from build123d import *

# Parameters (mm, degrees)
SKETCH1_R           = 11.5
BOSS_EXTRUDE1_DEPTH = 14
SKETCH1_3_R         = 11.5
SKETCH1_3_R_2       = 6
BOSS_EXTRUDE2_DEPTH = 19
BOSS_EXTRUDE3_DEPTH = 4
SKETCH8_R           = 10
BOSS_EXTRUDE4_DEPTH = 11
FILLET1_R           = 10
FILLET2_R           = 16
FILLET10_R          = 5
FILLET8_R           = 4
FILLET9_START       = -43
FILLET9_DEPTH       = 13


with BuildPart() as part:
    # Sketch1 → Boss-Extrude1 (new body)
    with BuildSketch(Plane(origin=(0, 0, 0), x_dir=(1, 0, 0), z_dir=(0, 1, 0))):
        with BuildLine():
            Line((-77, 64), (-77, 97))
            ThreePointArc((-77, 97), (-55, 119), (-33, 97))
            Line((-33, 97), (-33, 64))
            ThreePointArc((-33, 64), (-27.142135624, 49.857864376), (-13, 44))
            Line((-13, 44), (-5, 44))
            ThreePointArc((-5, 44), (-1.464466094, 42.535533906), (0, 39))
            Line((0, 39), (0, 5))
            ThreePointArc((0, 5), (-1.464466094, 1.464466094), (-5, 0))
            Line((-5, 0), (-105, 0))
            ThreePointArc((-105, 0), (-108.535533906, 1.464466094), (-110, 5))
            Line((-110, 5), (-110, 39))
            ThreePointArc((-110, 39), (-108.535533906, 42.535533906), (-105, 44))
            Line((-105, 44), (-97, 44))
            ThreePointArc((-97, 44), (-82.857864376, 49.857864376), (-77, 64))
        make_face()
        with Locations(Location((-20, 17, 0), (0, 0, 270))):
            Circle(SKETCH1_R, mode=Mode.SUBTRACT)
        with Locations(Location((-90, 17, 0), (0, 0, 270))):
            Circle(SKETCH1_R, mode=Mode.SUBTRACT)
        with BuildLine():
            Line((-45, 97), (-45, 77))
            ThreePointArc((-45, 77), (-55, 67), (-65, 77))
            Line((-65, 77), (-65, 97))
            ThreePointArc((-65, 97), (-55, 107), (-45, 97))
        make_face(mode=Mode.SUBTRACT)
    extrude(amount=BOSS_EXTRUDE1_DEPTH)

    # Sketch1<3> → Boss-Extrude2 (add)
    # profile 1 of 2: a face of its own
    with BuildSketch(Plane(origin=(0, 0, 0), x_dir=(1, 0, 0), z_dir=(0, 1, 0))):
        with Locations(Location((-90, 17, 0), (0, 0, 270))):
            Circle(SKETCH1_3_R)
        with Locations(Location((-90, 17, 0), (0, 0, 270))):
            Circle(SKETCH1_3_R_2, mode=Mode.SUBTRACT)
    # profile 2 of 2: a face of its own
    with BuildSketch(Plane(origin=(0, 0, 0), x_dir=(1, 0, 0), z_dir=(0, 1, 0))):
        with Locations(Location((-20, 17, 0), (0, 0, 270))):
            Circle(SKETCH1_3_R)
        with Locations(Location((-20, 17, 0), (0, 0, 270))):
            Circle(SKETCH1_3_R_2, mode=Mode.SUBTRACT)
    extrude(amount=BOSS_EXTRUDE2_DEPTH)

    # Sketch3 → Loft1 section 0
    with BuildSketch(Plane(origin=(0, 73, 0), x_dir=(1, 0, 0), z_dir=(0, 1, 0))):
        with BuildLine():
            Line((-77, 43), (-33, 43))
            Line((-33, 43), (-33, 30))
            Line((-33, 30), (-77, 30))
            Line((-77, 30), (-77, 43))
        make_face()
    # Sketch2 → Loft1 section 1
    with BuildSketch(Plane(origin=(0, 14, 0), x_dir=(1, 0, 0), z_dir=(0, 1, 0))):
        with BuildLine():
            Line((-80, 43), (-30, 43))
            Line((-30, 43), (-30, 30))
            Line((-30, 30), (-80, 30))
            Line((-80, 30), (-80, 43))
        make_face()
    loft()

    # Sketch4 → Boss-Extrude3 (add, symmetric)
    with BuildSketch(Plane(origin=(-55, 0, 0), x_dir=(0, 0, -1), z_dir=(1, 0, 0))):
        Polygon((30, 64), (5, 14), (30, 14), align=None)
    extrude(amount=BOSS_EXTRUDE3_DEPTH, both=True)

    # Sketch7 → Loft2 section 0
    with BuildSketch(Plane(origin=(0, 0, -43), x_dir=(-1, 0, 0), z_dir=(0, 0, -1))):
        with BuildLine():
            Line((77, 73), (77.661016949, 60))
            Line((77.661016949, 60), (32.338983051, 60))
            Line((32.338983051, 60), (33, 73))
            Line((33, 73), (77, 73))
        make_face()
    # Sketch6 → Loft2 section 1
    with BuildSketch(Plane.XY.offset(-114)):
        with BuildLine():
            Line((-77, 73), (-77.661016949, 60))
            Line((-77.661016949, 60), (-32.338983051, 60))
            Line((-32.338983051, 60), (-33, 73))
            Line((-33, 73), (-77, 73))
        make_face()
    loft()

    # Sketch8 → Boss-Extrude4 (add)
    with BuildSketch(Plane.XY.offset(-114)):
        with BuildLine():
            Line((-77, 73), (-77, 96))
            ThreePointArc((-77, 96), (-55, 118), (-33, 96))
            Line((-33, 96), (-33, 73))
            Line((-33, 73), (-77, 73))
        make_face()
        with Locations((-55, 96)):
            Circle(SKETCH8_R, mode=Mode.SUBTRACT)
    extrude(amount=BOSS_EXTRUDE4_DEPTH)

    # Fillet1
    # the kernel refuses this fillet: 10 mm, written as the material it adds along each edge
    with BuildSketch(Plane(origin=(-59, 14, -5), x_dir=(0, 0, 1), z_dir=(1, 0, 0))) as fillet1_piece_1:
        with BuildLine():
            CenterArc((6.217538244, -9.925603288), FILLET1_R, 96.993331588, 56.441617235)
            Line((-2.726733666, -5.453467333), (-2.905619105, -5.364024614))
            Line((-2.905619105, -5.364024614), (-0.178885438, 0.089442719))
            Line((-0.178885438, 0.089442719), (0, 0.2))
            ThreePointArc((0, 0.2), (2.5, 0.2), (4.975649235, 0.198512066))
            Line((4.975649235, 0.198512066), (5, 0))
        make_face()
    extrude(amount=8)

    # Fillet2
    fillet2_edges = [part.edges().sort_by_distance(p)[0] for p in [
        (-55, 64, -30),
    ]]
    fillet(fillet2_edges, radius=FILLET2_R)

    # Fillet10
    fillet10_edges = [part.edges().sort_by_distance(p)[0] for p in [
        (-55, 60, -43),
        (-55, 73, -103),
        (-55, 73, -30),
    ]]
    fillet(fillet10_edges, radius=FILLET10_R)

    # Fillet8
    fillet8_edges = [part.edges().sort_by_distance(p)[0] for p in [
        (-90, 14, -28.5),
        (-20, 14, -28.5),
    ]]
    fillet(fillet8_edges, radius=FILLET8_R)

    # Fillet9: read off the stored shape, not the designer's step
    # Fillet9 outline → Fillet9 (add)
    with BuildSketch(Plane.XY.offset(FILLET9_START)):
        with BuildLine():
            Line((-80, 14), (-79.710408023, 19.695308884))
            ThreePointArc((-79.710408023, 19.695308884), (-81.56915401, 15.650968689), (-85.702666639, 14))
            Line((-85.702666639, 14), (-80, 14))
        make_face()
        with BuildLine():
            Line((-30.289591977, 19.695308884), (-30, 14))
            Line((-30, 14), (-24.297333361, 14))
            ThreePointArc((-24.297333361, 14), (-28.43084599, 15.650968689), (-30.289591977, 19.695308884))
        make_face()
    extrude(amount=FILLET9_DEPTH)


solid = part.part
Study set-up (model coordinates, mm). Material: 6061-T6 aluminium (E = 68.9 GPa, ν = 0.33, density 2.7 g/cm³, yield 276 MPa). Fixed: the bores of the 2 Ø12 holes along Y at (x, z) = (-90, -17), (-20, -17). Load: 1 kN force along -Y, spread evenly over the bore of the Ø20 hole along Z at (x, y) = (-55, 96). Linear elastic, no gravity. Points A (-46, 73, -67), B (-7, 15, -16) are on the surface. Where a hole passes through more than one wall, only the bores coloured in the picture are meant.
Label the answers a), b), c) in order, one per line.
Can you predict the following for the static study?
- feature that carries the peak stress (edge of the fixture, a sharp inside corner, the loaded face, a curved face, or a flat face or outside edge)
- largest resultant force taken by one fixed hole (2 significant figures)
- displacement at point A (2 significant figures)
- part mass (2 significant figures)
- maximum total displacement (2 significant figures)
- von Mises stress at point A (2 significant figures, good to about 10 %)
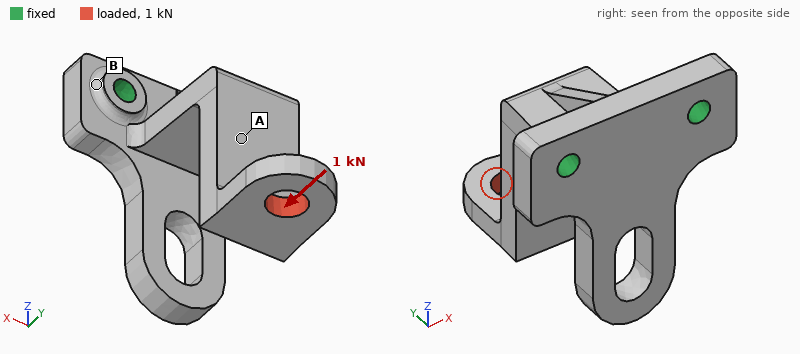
a) a curved face
b) 550 N
c) 0.22 mm
d) 550 g
e) 0.71 mm
f) 32 MPa
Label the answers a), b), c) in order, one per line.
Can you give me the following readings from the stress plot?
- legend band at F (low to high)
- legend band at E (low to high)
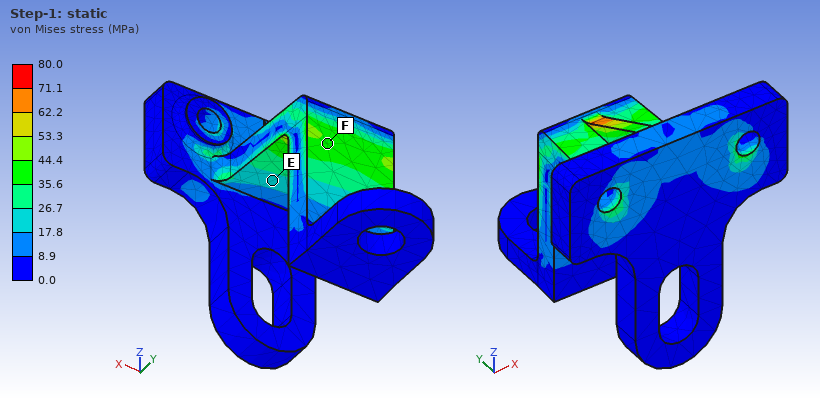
a) 35.6 to 44.4 MPa
b) 17.8 to 26.7 MPa
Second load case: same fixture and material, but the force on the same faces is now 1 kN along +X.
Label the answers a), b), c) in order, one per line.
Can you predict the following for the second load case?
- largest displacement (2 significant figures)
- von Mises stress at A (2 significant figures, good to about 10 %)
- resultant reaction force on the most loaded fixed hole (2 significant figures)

a) 0.40 mm
b) 23 MPa
c) 2.0 kN
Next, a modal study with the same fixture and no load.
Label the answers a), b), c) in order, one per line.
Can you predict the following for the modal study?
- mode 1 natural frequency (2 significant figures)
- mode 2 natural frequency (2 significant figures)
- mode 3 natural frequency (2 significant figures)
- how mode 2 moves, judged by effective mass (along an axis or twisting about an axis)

a) 670 Hz
b) 970 Hz
c) 1700 Hz
d) along X
